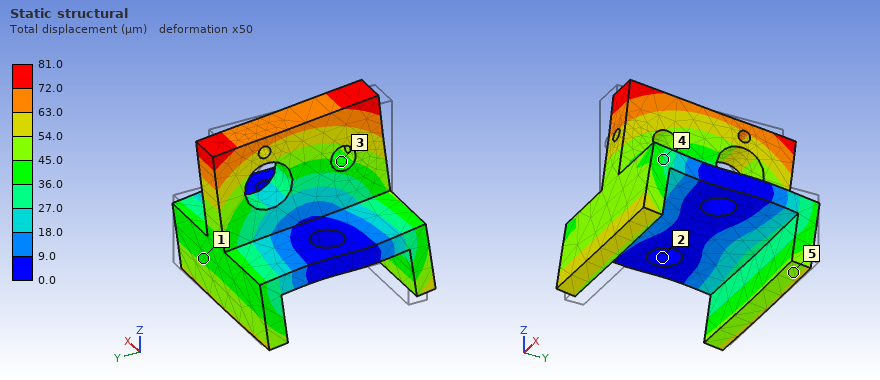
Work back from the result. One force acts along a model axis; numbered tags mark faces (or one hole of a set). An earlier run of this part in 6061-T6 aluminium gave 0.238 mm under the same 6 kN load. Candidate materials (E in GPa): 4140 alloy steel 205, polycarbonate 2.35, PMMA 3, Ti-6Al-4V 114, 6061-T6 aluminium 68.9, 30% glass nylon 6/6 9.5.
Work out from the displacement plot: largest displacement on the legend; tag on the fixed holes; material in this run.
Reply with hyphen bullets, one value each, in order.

- 81.0 µm
- 2
- 4140 alloy steel
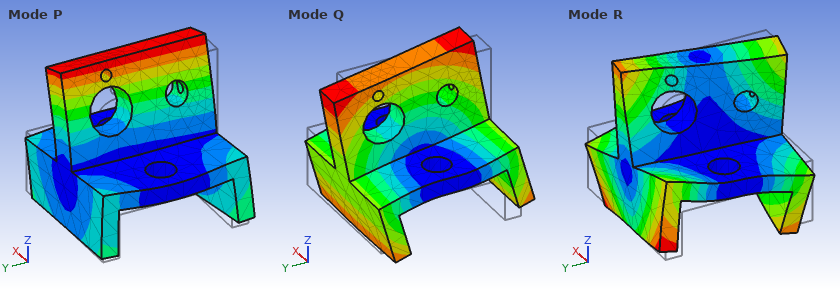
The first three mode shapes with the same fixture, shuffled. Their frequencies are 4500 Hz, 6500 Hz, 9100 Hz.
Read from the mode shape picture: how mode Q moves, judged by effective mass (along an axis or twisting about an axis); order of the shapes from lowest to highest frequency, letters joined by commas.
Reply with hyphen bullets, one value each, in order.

- twisting about X
- Q, P, R
